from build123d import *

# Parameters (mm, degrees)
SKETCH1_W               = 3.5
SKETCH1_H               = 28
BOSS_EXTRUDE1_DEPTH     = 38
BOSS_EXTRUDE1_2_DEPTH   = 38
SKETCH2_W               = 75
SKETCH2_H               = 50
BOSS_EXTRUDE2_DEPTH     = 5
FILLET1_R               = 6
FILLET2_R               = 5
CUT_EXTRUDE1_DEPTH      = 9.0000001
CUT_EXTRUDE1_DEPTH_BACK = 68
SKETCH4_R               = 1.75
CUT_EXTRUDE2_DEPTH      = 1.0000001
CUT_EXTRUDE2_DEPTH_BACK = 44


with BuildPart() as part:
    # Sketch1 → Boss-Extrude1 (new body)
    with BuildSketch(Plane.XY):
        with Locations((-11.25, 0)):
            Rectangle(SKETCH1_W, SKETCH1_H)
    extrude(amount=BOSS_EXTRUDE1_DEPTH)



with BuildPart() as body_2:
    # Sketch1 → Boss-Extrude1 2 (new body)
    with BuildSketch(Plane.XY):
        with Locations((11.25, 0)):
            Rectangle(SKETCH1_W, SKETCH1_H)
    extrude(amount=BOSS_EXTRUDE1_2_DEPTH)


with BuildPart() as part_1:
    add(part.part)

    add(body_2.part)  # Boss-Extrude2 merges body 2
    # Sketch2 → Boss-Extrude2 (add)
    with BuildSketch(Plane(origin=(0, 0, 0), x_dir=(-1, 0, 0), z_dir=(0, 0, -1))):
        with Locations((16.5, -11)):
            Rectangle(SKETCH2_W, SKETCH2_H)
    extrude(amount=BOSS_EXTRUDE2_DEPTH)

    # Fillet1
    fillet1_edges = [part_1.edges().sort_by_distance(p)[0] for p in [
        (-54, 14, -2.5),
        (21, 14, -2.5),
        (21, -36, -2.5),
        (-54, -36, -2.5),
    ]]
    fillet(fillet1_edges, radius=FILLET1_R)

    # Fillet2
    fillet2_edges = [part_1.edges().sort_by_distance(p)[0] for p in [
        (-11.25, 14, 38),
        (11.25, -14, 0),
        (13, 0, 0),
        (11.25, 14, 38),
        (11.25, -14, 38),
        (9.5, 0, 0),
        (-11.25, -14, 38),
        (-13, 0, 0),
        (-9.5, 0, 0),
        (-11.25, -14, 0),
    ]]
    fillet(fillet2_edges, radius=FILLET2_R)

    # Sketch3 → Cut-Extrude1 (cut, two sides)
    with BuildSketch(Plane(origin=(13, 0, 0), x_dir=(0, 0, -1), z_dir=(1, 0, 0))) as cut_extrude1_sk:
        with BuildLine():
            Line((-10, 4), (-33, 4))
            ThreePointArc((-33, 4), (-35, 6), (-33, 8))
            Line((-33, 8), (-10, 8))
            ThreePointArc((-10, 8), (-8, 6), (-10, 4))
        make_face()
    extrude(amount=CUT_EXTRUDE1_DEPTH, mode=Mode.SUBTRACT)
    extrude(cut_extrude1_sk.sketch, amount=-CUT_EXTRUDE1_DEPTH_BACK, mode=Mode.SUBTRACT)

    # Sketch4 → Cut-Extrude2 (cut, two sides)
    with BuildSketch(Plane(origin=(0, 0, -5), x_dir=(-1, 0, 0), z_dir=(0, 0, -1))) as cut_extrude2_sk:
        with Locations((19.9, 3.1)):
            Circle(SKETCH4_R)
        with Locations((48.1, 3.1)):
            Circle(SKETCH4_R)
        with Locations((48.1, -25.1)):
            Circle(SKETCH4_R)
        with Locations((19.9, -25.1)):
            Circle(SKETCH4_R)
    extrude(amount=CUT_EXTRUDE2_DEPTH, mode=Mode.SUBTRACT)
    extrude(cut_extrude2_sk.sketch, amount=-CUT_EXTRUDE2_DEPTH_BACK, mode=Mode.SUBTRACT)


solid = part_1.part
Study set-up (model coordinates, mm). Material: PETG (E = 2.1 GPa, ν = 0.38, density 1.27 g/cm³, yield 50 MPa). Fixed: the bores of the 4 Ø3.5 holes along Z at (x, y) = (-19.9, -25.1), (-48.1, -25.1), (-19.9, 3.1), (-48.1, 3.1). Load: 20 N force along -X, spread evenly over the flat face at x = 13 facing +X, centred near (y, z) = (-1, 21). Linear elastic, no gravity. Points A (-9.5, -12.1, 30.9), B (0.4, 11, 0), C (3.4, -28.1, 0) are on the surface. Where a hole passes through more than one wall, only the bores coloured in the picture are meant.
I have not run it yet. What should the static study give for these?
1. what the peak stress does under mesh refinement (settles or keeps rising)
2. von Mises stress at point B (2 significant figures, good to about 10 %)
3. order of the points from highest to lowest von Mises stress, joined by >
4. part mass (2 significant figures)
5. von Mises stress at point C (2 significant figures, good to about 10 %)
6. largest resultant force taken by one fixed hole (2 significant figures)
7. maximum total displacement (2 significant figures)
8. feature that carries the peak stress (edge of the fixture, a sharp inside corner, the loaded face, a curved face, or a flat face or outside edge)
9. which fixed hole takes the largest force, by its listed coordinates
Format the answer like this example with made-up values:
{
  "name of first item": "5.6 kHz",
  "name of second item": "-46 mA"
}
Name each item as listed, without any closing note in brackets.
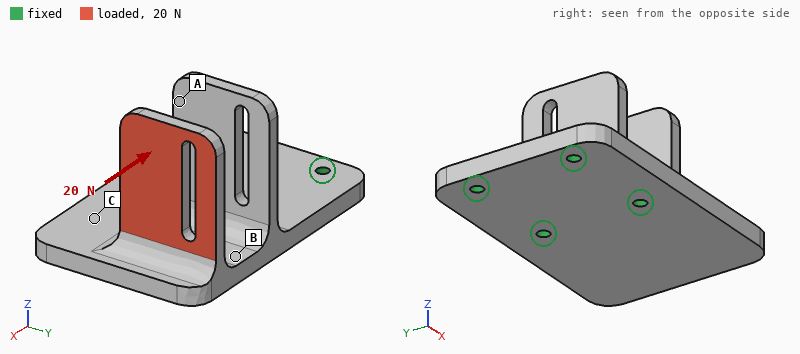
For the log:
{
  "what the peak stress does under mesh refinement": "keeps rising",
  "von Mises stress at point B": "2.8 MPa",
  "order of the points from highest to lowest von Mises stress, joined by >": "B > C > A",
  "part mass": "33 g",
  "von Mises stress at point C": "1.3 MPa",
  "largest resultant force taken by one fixed hole": "14 N",
  "maximum total displacement": "1.1 mm",
  "feature that carries the peak stress": "edge of the fixture",
  "which fixed hole takes the largest force, by its listed coordinates": "(-19.9, 3.1)"
}
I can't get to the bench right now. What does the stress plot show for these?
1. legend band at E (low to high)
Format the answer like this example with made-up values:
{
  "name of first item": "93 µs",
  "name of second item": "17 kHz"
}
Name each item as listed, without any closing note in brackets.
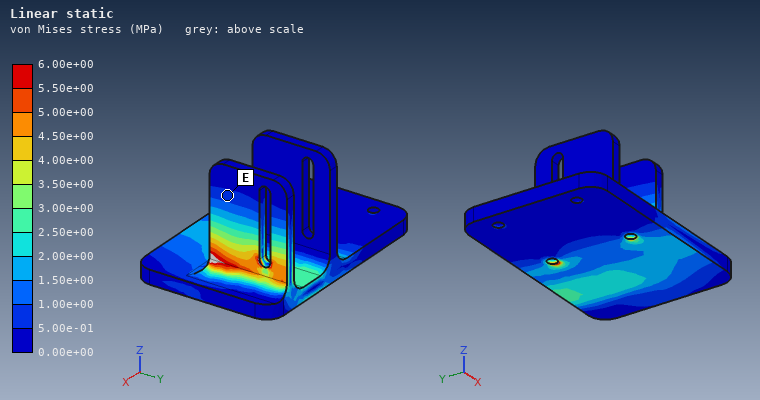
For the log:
{
  "legend band at E": "5.00e-01 to 1.00e+00 MPa"
}
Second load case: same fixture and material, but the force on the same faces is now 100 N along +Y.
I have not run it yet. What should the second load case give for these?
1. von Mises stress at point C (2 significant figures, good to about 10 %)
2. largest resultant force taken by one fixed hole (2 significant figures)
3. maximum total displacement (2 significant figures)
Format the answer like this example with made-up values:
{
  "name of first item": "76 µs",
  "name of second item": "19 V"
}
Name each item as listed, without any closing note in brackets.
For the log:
{
  "von Mises stress at point C": "3.4 MPa",
  "largest resultant force taken by one fixed hole": "130 N",
  "maximum total displacement": "1.2 mm"
}
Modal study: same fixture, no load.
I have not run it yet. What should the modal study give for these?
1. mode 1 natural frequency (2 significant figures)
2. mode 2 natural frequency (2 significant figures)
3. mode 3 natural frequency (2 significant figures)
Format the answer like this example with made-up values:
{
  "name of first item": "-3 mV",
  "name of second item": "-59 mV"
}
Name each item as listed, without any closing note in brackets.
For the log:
{
  "mode 1 natural frequency": "360 Hz",
  "mode 2 natural frequency": "550 Hz",
  "mode 3 natural frequency": "750 Hz"
}
